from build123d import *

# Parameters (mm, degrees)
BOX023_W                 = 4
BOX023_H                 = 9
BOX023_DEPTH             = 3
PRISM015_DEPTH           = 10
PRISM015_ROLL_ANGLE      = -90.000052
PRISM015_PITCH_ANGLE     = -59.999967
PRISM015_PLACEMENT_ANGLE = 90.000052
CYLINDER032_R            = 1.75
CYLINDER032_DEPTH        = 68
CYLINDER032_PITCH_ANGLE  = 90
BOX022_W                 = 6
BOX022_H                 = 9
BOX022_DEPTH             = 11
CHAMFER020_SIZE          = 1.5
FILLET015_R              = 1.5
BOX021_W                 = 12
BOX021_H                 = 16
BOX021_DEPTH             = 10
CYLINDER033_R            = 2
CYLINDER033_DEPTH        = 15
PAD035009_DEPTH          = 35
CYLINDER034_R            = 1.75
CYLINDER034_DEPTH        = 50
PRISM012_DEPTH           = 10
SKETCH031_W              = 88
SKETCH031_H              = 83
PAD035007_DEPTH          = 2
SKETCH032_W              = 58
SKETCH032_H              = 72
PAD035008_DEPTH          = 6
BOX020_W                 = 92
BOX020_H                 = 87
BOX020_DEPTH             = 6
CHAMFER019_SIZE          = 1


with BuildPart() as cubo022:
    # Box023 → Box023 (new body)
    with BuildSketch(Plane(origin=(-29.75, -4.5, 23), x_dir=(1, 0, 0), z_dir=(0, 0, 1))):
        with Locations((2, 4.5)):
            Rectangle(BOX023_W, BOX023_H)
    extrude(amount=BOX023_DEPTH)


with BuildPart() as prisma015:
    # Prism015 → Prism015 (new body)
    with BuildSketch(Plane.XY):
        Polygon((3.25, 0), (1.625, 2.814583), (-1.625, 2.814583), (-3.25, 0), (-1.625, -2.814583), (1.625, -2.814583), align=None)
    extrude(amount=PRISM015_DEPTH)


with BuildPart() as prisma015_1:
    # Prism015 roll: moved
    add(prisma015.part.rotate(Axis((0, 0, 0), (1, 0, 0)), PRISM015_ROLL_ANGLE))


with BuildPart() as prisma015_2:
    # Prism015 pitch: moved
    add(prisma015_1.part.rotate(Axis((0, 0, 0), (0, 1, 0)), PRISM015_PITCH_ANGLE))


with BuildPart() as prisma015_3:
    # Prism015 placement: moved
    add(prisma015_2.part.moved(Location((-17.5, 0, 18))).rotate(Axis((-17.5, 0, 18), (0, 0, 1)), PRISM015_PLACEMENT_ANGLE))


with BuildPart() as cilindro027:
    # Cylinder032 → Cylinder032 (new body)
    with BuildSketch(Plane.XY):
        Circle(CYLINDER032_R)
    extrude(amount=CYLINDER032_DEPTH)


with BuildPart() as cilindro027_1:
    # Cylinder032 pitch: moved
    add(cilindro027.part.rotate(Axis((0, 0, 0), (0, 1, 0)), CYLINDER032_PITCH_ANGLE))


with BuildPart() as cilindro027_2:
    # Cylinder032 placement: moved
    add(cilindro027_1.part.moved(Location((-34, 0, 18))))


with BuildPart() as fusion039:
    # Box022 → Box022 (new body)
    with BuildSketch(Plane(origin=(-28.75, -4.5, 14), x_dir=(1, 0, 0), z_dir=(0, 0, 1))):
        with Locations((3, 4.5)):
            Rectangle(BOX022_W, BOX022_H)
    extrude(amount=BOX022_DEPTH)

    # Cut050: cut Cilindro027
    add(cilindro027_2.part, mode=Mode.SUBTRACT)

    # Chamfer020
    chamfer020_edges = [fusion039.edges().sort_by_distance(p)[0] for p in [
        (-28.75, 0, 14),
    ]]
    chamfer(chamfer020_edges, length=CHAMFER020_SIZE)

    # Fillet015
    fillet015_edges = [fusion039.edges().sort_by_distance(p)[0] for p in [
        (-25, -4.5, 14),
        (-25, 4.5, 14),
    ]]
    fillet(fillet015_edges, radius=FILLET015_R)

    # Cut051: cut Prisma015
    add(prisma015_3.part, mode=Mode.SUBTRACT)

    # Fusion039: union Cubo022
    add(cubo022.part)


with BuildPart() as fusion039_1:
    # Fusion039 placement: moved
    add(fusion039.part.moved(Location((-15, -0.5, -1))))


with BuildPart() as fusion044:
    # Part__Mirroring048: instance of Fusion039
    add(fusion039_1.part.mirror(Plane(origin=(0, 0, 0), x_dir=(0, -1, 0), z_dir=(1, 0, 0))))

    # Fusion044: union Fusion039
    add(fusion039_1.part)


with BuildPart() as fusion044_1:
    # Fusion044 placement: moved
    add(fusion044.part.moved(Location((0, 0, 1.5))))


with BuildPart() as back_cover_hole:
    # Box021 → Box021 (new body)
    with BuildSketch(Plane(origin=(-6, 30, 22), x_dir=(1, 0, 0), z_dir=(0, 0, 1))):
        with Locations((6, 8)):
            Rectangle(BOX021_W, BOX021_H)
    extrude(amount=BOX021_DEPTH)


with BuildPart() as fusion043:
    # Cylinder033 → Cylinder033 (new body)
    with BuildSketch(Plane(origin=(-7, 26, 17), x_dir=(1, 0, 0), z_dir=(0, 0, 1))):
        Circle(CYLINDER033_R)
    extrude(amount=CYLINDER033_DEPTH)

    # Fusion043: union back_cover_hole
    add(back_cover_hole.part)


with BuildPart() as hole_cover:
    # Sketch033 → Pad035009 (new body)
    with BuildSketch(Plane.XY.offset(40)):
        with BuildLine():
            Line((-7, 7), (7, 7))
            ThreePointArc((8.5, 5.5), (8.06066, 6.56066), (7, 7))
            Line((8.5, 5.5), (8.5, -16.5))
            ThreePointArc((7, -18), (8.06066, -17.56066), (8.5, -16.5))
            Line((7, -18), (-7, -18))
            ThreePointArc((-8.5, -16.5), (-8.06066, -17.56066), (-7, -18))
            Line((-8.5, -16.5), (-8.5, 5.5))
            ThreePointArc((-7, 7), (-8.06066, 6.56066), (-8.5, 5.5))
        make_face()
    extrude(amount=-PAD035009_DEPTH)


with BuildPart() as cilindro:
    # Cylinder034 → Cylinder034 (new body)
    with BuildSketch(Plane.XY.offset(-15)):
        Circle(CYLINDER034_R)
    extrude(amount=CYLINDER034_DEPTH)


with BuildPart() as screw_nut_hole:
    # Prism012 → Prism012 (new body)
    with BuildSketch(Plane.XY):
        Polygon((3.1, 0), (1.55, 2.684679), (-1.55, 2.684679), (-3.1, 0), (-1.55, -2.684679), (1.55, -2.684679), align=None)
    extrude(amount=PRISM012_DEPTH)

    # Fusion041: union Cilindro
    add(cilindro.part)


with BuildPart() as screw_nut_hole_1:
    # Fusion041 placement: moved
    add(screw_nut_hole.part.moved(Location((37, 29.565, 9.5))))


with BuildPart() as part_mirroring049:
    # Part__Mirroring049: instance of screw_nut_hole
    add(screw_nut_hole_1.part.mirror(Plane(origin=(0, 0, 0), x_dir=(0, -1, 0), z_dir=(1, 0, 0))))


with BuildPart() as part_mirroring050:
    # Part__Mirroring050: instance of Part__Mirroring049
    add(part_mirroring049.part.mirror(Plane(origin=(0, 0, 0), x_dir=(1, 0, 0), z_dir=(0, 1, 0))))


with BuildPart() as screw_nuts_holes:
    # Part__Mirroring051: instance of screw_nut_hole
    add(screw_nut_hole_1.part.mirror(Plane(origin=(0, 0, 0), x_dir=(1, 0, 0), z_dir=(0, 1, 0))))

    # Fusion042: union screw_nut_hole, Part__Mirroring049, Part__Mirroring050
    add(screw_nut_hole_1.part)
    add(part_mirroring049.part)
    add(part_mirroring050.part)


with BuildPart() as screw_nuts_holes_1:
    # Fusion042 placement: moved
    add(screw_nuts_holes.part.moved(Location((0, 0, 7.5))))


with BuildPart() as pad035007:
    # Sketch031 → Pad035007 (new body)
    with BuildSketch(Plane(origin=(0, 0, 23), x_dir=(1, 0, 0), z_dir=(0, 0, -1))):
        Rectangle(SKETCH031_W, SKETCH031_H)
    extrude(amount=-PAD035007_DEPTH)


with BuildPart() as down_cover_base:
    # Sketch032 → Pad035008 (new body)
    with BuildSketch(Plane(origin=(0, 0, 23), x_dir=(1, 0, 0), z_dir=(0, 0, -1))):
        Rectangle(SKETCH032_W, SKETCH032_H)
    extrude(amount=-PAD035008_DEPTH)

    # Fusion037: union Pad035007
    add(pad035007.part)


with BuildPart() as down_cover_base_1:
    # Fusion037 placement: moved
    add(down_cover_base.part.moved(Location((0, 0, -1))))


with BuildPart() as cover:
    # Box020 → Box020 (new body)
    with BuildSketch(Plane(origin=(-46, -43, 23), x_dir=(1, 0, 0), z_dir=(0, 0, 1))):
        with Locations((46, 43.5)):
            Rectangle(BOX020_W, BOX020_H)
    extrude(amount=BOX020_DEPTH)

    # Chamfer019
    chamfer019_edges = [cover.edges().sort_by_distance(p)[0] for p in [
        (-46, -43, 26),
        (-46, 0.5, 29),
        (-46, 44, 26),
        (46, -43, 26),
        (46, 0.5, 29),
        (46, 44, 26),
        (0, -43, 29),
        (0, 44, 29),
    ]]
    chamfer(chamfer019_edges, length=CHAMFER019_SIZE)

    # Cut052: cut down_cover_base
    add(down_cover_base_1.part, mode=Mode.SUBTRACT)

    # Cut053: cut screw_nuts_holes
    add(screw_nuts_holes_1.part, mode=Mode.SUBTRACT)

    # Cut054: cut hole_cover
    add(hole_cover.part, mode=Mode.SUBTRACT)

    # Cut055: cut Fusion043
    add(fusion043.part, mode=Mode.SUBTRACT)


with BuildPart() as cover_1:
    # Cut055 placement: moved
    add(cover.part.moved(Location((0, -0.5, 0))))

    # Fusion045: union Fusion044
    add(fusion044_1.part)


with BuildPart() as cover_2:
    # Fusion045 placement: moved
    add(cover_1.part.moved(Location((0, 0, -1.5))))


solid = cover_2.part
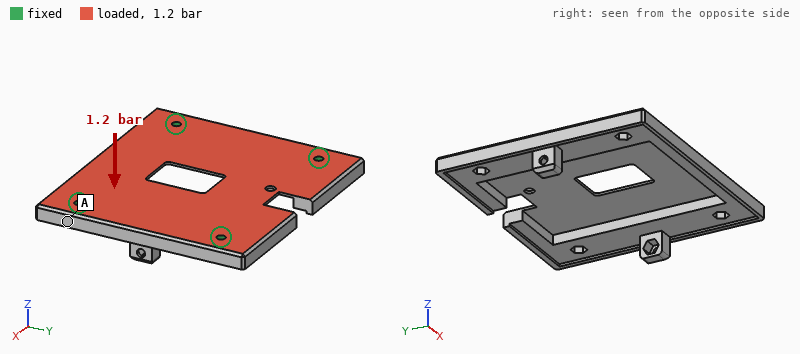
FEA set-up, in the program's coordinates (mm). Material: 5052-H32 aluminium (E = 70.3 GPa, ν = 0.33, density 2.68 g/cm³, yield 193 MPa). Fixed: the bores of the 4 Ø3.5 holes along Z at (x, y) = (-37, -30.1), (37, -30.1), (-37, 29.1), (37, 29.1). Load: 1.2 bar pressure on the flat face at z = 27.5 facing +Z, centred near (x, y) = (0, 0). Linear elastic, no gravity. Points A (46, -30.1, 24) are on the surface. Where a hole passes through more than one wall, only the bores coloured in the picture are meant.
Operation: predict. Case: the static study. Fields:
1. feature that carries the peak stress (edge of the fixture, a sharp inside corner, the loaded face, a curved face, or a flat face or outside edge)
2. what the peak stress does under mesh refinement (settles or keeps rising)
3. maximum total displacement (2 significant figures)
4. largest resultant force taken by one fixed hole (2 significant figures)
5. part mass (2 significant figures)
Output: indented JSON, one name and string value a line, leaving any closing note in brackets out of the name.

{
  "feature that carries the peak stress": "edge of the fixture",
  "what the peak stress does under mesh refinement": "keeps rising",
  "maximum total displacement": "0.49 mm",
  "largest resultant force taken by one fixed hole": "280 N",
  "part mass": "62 g"
}
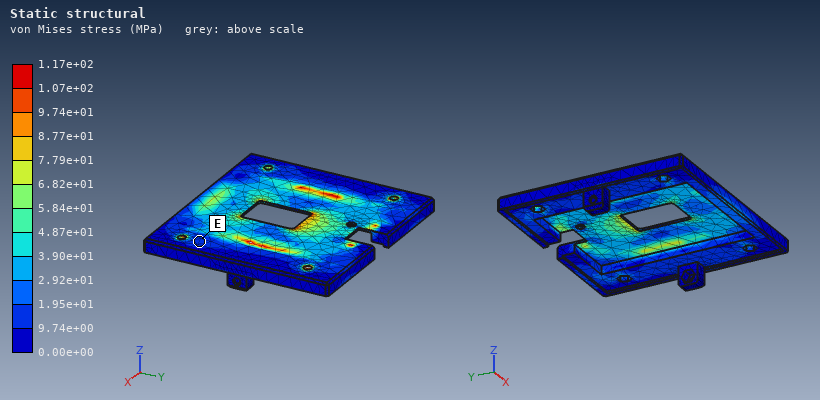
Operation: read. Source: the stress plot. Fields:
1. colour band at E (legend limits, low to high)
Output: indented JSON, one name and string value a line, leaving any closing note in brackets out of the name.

{
  "colour band at E": "9.74e+00 to 1.95e+01 MPa"
}
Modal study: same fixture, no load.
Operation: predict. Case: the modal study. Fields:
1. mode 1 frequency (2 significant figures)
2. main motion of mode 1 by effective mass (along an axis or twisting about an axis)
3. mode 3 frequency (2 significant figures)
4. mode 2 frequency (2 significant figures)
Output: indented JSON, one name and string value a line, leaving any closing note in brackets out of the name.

{
  "mode 1 frequency": "2100 Hz",
  "main motion of mode 1 by effective mass": "along Z",
  "mode 3 frequency": "3300 Hz",
  "mode 2 frequency": "3000 Hz"
}
